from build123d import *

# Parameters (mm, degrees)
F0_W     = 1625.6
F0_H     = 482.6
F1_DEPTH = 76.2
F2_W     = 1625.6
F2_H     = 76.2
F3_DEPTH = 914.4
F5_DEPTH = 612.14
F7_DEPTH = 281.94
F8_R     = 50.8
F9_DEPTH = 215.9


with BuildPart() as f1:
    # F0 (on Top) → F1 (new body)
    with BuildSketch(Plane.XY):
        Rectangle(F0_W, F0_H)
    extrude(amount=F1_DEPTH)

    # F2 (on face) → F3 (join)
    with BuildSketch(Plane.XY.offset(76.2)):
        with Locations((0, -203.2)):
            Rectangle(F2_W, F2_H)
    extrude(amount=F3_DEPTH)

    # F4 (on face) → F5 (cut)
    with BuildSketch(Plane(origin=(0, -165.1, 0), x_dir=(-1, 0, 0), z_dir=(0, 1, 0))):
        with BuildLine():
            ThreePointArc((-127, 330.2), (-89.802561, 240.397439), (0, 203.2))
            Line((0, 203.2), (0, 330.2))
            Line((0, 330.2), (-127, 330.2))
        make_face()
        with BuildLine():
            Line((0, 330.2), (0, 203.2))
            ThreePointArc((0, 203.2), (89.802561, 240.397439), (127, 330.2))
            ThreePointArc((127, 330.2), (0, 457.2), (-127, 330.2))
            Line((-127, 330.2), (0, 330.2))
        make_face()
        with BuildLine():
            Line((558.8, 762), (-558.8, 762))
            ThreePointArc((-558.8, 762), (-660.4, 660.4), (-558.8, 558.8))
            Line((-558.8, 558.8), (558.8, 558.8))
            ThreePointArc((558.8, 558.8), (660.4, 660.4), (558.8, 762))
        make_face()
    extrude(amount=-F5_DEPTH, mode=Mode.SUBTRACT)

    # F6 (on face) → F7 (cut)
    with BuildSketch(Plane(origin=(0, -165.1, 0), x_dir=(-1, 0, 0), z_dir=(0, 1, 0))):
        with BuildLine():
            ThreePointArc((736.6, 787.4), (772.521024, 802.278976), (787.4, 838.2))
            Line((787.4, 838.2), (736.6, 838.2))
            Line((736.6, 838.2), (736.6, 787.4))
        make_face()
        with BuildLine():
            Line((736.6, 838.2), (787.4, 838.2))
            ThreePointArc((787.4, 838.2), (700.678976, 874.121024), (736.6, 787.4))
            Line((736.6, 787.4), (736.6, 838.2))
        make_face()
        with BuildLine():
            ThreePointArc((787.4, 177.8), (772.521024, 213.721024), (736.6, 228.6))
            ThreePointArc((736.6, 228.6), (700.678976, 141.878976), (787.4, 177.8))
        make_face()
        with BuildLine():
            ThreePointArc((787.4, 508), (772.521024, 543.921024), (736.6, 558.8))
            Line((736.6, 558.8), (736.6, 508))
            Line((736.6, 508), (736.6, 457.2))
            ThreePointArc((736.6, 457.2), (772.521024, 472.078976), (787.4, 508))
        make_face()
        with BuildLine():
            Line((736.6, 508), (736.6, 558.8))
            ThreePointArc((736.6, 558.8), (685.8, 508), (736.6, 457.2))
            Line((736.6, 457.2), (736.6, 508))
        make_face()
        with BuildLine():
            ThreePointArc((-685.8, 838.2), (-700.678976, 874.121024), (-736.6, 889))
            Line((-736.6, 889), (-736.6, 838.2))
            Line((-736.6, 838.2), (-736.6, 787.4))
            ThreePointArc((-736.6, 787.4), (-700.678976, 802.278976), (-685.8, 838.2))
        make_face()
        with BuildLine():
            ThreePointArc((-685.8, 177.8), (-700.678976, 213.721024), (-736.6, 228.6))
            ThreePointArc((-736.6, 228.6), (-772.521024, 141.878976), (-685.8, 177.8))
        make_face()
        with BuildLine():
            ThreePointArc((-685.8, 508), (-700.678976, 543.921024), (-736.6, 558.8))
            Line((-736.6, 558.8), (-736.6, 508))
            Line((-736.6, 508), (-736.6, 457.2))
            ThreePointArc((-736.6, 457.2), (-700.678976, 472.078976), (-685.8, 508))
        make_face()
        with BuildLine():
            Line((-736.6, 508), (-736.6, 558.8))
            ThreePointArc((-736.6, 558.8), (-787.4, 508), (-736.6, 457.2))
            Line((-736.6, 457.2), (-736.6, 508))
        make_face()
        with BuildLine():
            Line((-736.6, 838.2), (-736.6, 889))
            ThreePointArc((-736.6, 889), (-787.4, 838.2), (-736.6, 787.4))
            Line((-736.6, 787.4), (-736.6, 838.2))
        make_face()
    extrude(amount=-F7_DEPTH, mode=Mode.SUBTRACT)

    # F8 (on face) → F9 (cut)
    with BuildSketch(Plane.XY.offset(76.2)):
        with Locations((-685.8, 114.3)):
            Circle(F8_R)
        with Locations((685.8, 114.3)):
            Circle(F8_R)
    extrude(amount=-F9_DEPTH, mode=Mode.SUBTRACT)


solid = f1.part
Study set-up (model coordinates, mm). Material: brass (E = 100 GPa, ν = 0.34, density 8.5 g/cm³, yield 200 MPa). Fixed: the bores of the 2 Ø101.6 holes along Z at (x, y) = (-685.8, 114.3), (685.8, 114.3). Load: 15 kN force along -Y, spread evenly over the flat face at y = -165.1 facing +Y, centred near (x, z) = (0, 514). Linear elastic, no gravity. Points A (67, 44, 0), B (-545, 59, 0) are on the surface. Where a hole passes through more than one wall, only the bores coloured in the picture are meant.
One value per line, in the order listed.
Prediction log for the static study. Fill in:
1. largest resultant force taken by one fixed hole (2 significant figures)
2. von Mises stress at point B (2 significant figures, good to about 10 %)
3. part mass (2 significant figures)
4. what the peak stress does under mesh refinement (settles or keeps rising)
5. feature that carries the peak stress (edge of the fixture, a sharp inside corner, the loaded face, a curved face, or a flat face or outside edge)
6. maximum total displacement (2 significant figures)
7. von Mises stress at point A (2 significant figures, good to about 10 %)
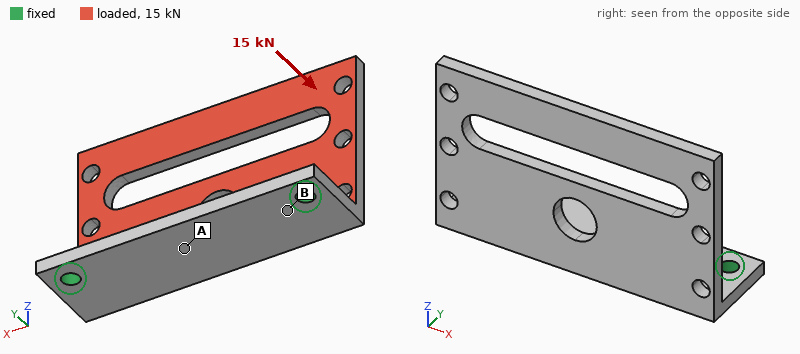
8.3 kN
4.6 MPa
1200 kg
keeps rising
edge of the fixture
1.1 mm
1.6 MPa
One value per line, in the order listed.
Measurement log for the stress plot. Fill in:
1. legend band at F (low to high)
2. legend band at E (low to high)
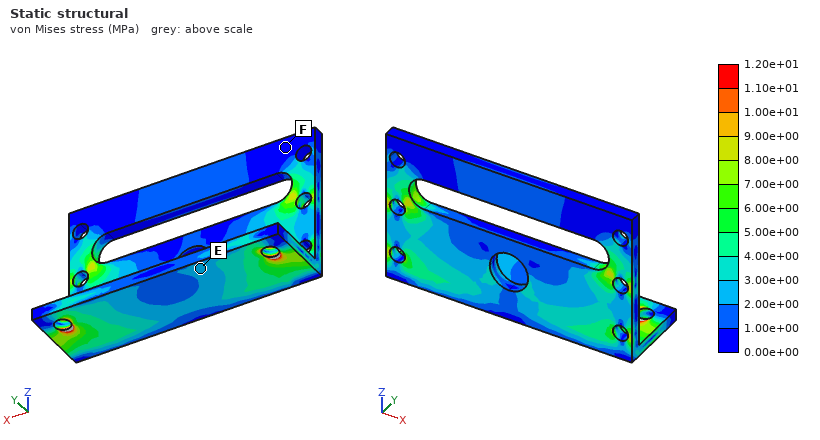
0.00e+00 to 1.00e+00 MPa
2.00e+00 to 3.00e+00 MPa
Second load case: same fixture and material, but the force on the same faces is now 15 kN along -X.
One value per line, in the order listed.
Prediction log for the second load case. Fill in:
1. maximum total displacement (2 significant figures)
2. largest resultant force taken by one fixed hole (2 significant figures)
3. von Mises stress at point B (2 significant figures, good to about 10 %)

91 µm
9.6 kN
1.0 MPa
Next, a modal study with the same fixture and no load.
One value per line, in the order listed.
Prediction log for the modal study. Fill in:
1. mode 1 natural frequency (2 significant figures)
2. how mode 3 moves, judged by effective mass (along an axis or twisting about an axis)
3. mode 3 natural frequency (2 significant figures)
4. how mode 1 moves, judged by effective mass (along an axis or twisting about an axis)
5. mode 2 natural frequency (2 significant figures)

27 Hz
along Z
91 Hz
along Y
60 Hz
